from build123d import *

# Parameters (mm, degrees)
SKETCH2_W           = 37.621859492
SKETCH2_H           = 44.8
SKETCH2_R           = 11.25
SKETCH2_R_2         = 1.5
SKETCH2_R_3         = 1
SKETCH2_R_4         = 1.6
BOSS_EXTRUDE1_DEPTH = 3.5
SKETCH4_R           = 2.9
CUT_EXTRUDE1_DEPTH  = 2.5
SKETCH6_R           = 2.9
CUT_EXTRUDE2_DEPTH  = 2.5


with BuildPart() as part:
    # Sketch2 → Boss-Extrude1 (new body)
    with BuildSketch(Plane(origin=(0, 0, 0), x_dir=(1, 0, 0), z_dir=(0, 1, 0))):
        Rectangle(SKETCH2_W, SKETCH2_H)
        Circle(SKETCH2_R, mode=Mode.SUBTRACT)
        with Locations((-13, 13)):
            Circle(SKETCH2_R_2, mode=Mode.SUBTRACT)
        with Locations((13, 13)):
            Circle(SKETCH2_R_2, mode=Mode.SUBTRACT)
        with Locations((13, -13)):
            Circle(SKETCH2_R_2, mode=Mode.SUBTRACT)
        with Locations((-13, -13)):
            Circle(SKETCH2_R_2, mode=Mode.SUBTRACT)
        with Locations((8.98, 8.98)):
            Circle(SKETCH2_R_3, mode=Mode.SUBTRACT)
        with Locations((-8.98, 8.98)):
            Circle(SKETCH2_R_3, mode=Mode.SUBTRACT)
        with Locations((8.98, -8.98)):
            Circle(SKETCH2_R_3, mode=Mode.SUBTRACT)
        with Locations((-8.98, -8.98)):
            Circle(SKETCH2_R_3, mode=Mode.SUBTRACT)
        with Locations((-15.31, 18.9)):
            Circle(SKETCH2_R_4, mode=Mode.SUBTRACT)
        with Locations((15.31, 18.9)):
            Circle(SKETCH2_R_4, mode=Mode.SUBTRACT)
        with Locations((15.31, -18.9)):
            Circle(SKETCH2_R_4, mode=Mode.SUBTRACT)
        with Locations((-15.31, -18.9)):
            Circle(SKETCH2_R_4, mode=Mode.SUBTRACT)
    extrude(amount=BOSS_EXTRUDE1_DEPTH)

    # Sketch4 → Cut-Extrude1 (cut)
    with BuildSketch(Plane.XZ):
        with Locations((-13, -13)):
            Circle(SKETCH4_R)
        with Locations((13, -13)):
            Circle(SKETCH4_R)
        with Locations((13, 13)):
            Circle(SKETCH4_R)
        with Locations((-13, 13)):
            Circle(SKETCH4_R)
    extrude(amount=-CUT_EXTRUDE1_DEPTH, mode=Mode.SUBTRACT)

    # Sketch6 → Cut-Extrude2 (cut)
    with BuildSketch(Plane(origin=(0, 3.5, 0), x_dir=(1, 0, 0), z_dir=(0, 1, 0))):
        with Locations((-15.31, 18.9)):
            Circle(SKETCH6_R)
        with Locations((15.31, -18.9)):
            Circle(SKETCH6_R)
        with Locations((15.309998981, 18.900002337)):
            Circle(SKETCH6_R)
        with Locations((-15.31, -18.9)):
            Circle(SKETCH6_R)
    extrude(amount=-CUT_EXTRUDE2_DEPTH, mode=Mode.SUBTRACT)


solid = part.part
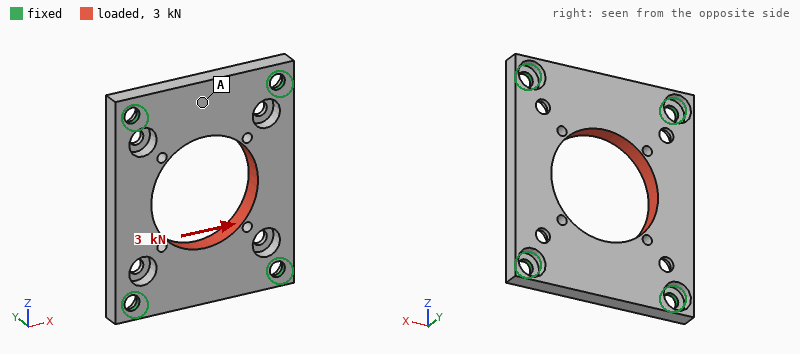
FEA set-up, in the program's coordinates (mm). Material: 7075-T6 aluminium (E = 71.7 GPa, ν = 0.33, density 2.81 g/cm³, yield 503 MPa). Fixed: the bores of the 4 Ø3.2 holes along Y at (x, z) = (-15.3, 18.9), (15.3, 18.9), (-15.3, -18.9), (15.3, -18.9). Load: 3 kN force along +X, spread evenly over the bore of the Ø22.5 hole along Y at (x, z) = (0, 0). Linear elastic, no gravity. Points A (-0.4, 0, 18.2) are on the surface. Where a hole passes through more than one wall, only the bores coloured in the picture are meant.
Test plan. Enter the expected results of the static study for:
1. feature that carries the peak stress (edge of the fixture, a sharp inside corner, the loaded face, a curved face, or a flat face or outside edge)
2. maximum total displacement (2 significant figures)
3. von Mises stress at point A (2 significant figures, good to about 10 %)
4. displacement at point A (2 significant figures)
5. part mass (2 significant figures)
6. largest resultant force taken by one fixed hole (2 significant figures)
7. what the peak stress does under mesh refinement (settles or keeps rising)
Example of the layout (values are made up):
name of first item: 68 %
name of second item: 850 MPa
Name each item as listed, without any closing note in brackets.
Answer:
feature that carries the peak stress: edge of the fixture
maximum total displacement: 20 µm
von Mises stress at point A: 20 MPa
displacement at point A: 8.2 µm
part mass: 11 g
largest resultant force taken by one fixed hole: 780 N
what the peak stress does under mesh refinement: keeps rising
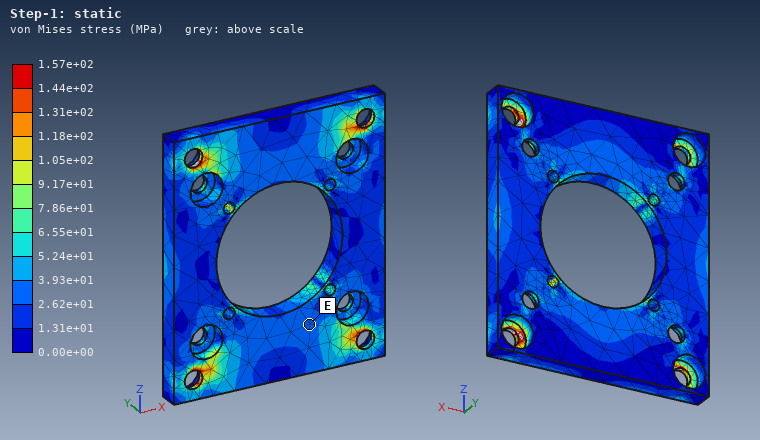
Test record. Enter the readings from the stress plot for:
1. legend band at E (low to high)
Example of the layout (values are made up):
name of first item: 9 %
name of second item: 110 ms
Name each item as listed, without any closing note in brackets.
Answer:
legend band at E: 2.62e+01 to 3.93e+01 MPa
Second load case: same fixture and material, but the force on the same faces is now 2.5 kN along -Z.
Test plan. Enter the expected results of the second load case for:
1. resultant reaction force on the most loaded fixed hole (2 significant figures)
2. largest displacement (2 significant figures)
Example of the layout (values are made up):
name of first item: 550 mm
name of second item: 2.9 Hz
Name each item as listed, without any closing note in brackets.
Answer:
resultant reaction force on the most loaded fixed hole: 640 N
largest displacement: 15 µm
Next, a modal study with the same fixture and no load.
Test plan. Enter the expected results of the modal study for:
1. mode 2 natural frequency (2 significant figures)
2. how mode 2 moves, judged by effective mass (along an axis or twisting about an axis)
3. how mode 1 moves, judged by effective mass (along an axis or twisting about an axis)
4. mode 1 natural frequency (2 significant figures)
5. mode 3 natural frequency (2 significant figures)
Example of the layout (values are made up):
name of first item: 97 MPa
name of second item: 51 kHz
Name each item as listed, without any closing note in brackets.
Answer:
mode 2 natural frequency: 11 kHz
how mode 2 moves, judged by effective mass: twisting about Z
how mode 1 moves, judged by effective mass: along Y
mode 1 natural frequency: 8200 Hz
mode 3 natural frequency: 13 kHz
